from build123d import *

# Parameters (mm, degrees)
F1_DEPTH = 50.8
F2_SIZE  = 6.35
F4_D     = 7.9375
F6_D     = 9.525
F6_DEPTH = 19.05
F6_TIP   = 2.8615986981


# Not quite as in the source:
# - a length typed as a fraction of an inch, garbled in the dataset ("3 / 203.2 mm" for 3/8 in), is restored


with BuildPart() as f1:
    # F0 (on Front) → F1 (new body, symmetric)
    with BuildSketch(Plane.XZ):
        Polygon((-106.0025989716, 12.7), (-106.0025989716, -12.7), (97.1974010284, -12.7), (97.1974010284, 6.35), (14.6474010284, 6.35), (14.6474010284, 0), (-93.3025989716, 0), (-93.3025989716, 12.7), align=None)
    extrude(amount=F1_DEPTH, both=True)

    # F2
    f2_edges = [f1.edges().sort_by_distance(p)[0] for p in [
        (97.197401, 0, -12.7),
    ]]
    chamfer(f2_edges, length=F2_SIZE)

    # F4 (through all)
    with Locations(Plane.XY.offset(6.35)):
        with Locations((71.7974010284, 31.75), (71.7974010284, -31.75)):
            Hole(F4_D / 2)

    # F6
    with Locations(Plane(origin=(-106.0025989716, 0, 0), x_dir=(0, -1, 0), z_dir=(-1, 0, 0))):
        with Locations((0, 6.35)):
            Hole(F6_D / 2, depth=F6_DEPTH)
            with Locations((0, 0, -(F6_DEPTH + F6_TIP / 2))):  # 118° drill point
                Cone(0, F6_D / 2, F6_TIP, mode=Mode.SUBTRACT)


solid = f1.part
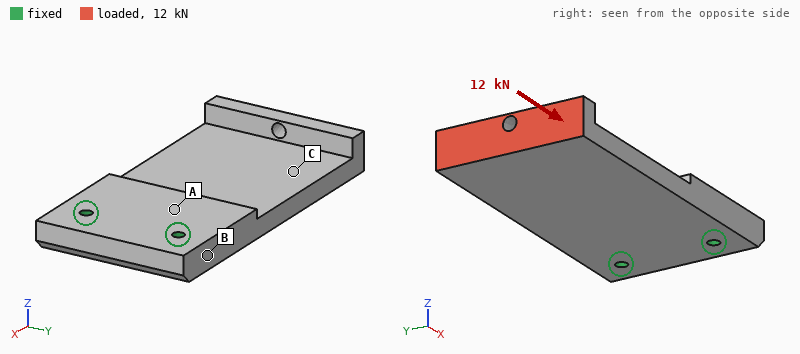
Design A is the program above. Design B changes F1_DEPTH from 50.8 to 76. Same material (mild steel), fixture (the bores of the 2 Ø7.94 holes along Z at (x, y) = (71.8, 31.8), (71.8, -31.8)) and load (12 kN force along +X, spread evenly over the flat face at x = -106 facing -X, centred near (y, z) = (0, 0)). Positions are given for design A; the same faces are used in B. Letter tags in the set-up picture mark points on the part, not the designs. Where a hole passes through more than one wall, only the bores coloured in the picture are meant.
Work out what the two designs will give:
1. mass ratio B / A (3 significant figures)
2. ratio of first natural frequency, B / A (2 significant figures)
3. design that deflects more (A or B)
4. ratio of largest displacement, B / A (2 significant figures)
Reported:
1.50
0.97
A
0.68
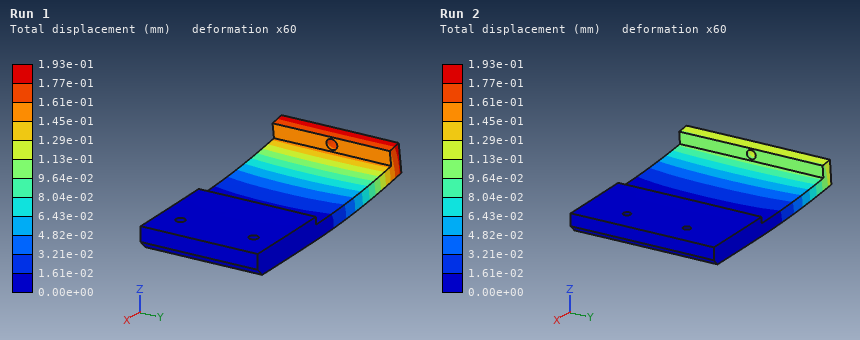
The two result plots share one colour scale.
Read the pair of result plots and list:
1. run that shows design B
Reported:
Run 2
